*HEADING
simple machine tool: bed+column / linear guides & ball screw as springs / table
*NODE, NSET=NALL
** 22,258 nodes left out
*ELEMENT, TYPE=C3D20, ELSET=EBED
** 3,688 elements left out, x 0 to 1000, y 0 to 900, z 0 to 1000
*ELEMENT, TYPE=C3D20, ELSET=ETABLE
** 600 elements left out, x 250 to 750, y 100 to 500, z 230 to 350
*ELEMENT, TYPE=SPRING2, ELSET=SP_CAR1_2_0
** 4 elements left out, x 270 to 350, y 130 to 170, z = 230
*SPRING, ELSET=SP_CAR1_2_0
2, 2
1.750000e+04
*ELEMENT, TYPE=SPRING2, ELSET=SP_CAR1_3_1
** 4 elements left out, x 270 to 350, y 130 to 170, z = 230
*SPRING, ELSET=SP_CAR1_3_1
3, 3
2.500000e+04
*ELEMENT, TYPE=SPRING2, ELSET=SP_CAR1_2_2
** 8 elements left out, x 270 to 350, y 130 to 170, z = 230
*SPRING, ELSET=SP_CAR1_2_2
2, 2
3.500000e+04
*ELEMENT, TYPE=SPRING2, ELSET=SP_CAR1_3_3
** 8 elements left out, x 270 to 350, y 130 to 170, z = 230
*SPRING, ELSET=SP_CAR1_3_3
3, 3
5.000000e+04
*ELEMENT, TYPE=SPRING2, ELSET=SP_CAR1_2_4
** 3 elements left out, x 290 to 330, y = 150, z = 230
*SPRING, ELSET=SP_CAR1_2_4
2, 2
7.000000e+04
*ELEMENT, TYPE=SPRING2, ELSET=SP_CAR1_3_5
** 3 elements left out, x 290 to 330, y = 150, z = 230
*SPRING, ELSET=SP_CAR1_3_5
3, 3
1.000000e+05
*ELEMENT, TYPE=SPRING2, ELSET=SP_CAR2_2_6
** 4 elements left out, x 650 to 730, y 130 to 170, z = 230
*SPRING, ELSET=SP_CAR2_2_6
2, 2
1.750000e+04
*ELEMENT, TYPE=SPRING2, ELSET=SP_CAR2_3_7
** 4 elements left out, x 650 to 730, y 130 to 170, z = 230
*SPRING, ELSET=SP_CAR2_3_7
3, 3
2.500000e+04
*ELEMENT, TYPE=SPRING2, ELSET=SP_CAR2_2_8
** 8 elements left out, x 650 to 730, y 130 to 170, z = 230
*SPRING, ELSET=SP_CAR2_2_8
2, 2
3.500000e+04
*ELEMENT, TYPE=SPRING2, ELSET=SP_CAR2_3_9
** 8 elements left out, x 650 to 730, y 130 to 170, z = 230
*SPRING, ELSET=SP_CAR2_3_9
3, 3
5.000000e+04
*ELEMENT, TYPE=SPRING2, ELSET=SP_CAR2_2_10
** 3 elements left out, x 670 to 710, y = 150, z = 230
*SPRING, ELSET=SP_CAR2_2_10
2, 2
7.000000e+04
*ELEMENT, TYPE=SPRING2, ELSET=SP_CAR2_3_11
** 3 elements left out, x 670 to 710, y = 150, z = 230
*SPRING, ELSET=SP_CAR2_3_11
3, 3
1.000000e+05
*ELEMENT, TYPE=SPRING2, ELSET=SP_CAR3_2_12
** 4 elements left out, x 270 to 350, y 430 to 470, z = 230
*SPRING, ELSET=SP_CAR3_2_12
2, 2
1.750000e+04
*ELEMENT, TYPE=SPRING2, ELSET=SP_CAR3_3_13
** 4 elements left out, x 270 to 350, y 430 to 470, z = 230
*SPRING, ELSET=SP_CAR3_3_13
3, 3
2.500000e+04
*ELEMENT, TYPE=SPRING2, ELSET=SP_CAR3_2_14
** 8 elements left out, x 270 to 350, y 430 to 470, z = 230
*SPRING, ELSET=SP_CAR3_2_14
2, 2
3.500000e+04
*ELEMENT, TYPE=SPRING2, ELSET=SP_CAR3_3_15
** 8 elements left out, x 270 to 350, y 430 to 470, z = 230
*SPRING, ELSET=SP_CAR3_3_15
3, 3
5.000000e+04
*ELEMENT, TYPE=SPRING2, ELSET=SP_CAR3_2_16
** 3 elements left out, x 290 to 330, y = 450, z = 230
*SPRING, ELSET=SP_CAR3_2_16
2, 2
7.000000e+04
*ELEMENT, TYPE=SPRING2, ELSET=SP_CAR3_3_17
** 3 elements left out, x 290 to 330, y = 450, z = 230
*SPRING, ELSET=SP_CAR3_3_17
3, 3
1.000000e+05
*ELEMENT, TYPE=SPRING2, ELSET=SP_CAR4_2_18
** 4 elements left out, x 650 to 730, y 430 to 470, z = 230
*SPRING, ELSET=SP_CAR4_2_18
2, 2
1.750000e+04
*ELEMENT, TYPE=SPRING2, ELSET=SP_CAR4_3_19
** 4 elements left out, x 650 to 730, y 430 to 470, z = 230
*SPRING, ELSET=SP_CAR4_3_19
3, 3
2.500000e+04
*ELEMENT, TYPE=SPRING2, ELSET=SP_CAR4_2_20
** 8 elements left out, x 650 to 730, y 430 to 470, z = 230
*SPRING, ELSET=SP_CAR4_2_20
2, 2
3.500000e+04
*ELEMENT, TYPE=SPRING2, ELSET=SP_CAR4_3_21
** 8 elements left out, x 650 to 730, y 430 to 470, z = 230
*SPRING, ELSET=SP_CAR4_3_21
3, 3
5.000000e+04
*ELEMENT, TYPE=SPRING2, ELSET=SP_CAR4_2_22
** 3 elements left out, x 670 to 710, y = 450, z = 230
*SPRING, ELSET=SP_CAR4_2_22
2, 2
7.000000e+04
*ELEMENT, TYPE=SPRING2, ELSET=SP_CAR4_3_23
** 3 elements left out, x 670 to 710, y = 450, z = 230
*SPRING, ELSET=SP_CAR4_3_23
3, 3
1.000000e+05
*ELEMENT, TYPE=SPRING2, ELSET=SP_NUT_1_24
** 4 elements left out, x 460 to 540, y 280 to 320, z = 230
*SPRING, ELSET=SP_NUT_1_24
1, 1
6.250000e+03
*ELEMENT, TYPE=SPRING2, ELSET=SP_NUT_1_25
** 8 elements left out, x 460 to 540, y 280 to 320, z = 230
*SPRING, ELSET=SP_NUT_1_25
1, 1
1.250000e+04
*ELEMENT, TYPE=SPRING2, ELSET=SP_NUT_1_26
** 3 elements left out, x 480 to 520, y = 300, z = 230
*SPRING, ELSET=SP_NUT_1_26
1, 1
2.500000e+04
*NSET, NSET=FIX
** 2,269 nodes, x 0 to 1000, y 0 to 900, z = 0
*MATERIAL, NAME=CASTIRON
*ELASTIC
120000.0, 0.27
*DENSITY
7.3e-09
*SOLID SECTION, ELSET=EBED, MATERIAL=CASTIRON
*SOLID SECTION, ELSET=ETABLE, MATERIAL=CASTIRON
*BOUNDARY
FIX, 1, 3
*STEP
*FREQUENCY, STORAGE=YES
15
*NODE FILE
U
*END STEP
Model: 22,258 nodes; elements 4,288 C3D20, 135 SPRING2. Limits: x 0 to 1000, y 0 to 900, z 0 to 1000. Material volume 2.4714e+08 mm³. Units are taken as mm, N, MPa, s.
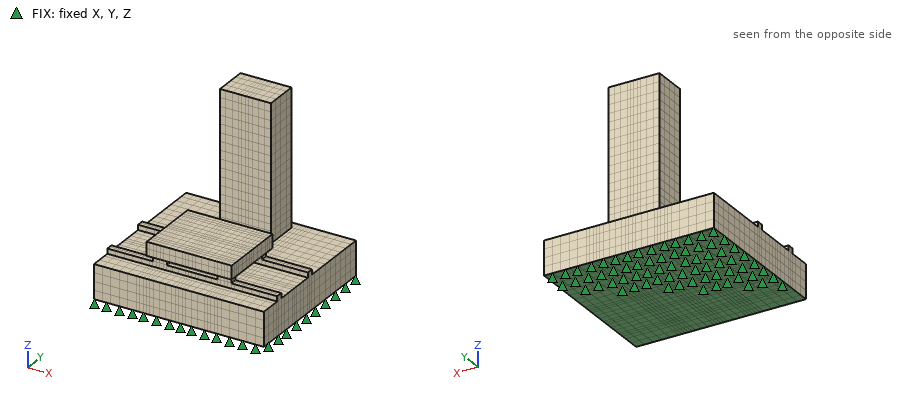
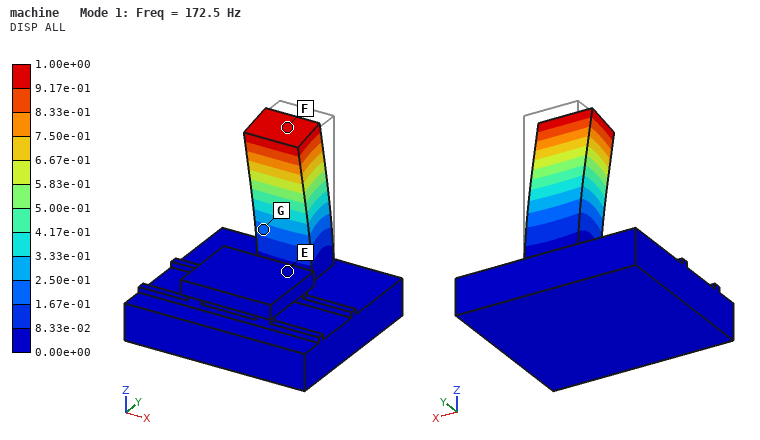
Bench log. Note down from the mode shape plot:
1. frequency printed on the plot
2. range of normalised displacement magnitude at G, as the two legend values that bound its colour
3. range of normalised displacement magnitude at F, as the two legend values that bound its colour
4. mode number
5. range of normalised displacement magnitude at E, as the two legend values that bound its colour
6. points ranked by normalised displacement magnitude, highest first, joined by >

172.5 Hz
1.67e-01 to 2.50e-01
9.17e-01 to 1.00e+00
1
0.00e+00 to 8.33e-02
F > G > E
